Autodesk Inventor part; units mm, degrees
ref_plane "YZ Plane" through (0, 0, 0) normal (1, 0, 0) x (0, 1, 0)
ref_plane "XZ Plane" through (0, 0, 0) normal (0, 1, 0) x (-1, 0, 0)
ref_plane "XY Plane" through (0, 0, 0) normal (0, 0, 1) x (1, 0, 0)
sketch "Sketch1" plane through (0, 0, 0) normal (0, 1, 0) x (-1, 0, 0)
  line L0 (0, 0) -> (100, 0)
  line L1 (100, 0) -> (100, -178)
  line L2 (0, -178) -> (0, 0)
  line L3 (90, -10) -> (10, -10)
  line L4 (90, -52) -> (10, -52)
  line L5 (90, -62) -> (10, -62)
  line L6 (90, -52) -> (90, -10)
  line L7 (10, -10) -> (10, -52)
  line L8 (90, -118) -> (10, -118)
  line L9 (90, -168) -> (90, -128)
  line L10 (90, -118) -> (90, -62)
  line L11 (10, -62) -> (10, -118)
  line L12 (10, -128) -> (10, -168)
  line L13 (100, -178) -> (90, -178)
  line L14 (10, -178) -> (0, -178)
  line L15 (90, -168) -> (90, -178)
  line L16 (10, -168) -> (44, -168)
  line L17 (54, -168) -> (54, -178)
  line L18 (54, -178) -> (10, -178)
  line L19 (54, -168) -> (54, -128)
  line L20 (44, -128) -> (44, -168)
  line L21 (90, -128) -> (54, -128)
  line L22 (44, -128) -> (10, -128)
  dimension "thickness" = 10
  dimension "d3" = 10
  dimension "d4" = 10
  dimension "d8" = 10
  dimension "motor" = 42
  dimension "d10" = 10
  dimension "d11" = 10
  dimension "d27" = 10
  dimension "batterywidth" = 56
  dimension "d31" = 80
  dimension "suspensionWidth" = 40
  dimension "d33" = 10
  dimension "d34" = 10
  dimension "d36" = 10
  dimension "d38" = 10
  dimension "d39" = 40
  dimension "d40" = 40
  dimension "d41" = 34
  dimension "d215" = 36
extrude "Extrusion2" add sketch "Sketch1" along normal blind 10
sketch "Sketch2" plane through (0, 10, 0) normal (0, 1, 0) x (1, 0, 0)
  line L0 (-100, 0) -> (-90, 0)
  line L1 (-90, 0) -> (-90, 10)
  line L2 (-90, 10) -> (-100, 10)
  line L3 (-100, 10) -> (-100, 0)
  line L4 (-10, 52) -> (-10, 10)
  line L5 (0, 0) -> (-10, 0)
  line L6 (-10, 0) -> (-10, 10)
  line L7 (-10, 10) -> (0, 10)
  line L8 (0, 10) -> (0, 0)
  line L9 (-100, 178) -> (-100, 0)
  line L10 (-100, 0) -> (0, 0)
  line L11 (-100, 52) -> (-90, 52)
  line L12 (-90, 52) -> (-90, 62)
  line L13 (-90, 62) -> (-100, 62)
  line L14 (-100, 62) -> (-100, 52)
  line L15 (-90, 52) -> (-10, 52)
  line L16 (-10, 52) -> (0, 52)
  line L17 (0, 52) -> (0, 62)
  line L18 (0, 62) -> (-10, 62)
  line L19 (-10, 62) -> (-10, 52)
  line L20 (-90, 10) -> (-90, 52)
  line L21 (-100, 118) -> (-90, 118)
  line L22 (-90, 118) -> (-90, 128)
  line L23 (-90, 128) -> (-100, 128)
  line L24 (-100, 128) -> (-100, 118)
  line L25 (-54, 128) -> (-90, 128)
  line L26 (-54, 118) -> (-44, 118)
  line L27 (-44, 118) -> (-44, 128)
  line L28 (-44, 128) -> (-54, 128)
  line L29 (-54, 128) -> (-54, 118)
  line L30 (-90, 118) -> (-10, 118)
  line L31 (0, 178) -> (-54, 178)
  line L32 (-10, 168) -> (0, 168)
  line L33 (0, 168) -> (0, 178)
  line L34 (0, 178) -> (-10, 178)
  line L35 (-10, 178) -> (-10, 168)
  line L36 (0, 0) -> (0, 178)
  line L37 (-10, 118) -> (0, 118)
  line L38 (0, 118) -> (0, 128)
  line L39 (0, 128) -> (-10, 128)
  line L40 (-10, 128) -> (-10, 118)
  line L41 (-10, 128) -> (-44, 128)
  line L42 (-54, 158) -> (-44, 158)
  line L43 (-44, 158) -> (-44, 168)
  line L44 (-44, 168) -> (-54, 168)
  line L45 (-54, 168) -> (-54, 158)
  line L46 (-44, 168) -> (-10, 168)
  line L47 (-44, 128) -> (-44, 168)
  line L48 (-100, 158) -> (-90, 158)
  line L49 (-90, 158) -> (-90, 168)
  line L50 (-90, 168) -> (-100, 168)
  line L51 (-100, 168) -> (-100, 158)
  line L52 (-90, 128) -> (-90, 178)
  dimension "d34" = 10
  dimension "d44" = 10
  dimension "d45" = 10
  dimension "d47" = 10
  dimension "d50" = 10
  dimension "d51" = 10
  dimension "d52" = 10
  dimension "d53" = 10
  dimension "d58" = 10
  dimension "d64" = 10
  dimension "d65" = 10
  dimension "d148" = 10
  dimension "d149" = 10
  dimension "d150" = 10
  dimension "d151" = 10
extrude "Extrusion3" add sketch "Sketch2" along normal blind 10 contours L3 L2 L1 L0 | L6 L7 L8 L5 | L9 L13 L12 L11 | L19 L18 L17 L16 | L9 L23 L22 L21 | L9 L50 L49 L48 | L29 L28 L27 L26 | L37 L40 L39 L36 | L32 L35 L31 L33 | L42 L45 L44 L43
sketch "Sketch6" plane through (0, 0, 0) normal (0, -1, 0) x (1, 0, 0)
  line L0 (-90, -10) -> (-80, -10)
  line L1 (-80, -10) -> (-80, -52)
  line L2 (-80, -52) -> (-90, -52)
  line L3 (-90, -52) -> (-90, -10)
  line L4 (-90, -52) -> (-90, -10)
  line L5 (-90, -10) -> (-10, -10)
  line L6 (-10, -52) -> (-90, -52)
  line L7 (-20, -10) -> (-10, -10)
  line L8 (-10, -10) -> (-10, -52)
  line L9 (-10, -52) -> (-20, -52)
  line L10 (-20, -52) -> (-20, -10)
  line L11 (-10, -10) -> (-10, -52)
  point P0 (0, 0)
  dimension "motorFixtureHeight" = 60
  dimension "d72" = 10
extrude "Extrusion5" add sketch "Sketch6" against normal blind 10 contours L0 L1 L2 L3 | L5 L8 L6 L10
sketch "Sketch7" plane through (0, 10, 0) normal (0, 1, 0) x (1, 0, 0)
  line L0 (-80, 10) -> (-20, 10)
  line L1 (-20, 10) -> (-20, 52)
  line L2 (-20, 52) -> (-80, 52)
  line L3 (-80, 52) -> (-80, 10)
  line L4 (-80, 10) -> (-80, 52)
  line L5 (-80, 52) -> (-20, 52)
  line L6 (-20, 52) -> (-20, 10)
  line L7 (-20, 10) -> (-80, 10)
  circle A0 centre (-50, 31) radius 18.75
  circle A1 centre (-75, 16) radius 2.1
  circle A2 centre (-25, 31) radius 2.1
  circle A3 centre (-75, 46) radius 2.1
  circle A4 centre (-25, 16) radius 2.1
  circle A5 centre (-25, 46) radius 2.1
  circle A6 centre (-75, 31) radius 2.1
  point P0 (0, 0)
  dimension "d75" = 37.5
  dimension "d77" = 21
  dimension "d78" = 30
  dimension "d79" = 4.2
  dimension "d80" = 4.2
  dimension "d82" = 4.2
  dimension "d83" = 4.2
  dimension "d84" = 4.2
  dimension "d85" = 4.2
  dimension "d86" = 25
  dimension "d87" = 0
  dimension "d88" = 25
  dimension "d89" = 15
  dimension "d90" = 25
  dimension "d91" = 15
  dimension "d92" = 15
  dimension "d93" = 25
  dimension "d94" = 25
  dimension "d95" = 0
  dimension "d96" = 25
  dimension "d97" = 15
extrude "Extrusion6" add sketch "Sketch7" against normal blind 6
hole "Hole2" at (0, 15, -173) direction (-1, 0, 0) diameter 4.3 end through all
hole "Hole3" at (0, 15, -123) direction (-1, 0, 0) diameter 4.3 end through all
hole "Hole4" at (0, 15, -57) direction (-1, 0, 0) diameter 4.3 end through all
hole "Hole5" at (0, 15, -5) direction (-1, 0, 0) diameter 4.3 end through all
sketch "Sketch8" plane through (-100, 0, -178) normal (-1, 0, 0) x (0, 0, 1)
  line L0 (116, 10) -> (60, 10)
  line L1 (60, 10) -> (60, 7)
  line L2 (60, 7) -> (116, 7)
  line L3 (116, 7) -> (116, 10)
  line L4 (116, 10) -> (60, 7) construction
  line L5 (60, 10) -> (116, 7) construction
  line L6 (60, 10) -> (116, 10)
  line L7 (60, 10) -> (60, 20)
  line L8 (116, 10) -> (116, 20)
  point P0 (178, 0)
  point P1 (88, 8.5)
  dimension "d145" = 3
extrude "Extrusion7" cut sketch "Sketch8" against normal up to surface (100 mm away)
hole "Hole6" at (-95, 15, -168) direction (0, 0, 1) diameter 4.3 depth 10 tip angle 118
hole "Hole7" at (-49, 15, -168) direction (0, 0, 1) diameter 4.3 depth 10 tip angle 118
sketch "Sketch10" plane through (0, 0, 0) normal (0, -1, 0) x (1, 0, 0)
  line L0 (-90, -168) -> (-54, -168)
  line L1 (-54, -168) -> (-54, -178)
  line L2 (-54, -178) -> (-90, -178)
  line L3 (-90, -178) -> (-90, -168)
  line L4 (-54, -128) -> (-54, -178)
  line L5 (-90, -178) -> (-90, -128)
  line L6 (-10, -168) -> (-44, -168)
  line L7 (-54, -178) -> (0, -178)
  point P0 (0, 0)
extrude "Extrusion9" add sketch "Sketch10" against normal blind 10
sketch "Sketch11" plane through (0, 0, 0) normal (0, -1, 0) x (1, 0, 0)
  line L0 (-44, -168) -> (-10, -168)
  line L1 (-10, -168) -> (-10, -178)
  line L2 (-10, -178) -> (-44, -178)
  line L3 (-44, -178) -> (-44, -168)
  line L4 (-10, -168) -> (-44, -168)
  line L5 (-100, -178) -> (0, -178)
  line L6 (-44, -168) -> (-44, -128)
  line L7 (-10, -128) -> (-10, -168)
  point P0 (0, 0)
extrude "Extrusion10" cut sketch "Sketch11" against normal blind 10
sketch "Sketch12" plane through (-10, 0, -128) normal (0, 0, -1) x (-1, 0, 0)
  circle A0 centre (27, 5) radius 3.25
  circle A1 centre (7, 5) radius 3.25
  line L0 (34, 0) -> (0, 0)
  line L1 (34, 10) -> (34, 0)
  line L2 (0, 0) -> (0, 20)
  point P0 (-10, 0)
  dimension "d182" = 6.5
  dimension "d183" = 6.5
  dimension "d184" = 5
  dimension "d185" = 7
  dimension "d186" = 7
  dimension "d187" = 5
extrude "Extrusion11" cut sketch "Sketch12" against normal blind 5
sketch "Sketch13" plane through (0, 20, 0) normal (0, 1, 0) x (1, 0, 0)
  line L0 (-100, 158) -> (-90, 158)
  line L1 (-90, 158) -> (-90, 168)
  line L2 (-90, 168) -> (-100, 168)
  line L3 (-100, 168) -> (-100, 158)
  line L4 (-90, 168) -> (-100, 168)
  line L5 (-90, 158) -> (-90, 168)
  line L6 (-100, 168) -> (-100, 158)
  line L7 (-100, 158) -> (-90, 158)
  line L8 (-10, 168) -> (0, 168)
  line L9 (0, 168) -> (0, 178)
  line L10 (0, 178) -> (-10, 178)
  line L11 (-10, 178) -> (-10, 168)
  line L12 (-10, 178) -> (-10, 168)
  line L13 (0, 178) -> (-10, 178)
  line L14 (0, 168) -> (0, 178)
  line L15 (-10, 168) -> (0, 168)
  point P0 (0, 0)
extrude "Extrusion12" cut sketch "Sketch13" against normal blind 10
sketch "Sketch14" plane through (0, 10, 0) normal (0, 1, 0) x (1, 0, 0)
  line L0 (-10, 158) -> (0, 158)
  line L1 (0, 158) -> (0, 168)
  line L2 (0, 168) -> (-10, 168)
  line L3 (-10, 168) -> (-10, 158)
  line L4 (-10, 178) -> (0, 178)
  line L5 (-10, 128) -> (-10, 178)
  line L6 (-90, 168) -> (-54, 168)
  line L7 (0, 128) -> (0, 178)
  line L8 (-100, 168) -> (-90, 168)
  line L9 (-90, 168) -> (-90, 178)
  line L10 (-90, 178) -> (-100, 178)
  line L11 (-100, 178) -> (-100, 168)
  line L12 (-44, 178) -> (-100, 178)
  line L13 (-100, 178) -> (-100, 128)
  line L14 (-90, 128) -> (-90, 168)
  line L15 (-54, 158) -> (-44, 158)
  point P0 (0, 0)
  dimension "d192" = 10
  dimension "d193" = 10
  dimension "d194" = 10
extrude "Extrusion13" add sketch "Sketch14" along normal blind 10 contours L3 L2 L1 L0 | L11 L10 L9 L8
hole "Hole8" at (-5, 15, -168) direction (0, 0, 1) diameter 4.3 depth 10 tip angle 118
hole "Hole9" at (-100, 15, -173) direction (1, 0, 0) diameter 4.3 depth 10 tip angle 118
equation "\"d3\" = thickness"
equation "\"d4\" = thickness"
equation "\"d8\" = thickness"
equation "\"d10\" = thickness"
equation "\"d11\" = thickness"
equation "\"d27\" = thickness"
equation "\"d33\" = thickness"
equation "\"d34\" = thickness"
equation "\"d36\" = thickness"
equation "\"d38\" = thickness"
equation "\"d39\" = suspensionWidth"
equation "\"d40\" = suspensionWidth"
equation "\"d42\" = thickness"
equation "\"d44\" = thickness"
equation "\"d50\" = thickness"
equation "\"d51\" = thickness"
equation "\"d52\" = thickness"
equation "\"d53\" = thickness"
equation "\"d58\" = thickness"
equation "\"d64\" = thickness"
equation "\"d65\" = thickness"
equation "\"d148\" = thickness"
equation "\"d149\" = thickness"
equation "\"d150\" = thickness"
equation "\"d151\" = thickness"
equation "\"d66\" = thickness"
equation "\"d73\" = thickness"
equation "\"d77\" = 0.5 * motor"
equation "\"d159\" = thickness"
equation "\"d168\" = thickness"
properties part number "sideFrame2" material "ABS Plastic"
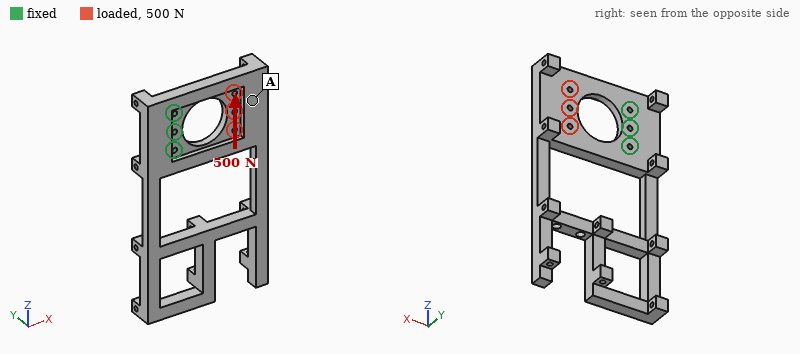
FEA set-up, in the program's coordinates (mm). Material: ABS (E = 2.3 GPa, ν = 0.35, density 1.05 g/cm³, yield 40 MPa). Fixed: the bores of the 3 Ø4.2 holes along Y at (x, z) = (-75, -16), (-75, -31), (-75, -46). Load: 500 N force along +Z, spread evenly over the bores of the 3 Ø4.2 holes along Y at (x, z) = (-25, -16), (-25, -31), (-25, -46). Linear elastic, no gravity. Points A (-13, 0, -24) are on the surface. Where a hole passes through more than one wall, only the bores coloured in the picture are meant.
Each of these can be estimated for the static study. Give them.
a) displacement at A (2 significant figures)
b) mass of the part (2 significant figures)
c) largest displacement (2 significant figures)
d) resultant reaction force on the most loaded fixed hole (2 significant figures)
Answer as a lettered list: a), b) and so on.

a) 0.81 mm
b) 94 g
c) 1.5 mm
d) 740 N
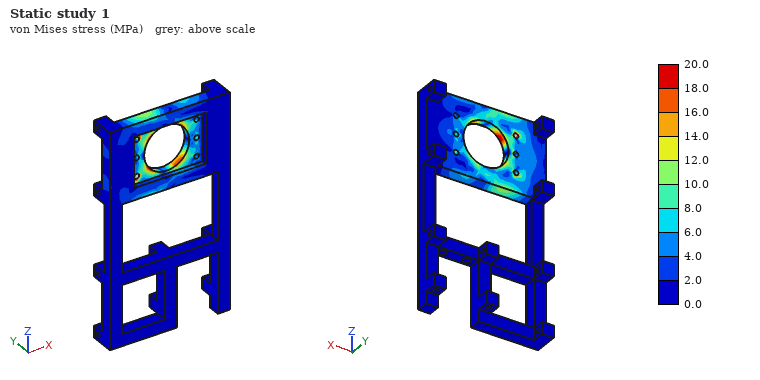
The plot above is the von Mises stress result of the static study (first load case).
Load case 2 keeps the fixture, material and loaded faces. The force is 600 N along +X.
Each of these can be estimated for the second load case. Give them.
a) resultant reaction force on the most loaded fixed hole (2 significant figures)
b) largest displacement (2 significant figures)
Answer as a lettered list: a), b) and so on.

a) 310 N
b) 0.49 mm
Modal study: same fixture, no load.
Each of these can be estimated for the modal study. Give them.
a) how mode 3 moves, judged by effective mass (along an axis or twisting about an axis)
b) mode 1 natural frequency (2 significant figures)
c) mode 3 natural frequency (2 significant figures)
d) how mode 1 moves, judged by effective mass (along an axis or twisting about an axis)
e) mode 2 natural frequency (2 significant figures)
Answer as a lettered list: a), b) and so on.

a) along X
b) 55 Hz
c) 200 Hz
d) along Y
e) 130 Hz
